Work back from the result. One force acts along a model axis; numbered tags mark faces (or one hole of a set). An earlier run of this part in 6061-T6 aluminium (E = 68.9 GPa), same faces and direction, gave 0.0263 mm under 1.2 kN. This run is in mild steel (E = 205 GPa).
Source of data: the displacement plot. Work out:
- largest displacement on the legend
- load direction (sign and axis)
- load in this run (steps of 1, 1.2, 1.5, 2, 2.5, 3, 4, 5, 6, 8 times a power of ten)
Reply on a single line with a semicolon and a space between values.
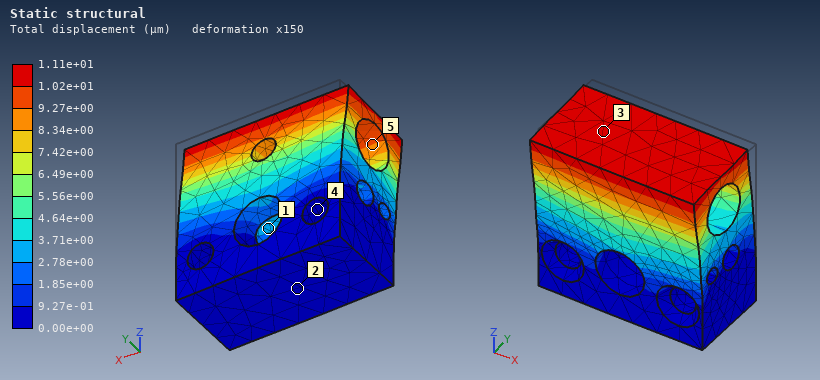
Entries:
1.11e+01 µm; -Y; 1.5 kN
